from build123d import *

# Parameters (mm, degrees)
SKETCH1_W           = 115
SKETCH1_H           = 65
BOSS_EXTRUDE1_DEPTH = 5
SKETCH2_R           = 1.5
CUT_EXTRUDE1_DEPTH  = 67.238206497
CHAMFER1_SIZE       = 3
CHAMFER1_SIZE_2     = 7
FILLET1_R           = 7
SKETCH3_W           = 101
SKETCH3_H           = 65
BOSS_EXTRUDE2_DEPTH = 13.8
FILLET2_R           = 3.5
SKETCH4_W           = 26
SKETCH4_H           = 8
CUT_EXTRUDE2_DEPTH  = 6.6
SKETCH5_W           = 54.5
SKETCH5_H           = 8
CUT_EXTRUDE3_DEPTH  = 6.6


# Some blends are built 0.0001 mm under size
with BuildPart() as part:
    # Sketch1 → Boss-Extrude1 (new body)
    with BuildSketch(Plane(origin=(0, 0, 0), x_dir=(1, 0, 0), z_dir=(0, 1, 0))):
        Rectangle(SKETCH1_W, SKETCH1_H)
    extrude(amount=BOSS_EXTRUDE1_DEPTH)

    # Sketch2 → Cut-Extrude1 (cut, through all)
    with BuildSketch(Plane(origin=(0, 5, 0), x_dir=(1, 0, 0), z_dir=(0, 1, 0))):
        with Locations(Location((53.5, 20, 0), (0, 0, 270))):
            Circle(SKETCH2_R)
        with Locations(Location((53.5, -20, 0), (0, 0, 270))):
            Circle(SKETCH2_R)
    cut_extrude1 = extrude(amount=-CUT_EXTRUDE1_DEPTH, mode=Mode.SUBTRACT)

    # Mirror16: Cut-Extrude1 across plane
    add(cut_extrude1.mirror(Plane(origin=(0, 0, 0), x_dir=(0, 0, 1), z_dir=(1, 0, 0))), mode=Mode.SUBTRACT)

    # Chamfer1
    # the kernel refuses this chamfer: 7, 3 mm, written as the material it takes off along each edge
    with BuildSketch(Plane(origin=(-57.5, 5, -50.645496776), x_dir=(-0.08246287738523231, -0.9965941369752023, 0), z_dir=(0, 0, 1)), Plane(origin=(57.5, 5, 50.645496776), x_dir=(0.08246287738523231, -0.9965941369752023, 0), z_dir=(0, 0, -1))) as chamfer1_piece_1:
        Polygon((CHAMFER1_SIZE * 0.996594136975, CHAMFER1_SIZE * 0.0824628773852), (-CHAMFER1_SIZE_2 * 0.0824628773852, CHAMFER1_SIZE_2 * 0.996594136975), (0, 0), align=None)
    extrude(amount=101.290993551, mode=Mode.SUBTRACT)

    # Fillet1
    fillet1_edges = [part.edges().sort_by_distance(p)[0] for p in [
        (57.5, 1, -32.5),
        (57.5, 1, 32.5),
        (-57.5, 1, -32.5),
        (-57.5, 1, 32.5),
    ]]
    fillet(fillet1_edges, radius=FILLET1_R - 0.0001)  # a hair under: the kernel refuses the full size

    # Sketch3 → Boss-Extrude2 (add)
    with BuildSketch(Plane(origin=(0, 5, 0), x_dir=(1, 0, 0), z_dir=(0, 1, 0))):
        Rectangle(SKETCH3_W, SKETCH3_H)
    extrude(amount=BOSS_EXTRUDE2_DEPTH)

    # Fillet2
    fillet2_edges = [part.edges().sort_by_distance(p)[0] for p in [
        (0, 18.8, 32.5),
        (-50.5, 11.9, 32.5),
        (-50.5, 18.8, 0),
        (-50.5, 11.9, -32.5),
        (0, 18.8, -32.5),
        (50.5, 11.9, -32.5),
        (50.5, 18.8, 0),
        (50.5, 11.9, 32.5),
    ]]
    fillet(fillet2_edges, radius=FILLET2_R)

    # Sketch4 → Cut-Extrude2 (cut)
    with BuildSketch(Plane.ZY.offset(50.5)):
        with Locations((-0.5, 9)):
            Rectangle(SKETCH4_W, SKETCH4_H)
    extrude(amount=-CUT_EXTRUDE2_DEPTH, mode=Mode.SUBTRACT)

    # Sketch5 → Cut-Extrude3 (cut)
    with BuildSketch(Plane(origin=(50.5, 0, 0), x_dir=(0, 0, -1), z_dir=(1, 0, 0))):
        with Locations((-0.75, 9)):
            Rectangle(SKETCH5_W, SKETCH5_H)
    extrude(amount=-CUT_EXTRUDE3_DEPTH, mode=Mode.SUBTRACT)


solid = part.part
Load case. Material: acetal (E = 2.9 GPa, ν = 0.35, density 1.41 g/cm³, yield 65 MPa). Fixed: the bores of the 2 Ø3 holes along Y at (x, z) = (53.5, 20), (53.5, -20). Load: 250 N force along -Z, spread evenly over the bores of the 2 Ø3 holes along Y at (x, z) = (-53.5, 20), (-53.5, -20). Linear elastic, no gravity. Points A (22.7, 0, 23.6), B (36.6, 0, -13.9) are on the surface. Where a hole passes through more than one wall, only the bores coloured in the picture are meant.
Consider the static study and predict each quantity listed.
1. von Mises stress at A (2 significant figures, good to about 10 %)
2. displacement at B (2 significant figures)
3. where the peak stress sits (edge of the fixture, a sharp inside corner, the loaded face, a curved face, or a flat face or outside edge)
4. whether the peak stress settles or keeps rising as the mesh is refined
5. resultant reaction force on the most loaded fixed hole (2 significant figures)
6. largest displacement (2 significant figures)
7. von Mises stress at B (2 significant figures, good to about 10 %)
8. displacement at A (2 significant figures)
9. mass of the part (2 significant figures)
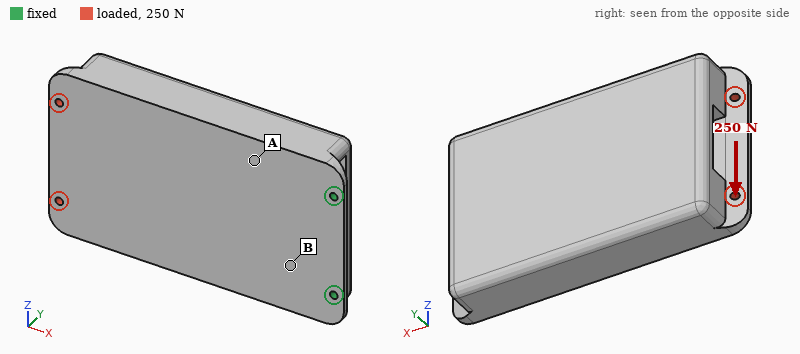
2.5 MPa
0.081 mm
edge of the fixture
keeps rising
660 N
0.52 mm
5.0 MPa
0.17 mm
170 g
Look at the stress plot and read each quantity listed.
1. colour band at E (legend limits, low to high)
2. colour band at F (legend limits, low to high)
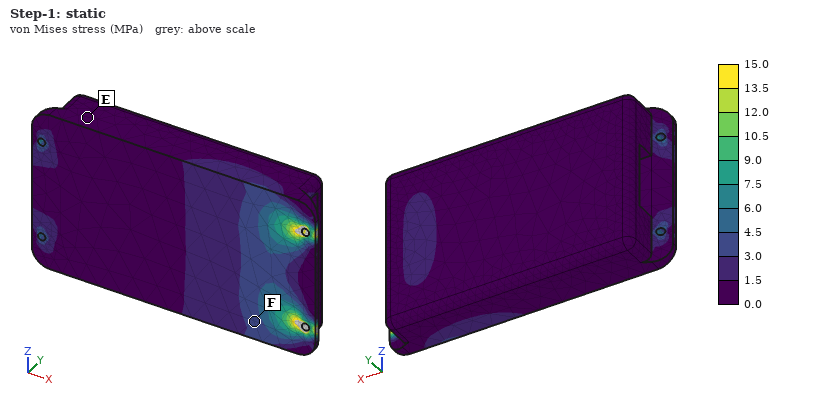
0.0 to 1.5 MPa
3.0 to 4.5 MPa
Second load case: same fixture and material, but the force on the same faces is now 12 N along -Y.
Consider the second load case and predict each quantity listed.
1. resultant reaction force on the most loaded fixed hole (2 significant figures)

10 N
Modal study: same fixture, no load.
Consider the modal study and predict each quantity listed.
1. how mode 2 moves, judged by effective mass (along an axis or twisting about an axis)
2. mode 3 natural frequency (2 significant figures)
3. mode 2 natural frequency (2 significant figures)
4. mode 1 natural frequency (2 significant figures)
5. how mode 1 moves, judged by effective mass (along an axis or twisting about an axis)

along Z
680 Hz
500 Hz
61 Hz
along Y
